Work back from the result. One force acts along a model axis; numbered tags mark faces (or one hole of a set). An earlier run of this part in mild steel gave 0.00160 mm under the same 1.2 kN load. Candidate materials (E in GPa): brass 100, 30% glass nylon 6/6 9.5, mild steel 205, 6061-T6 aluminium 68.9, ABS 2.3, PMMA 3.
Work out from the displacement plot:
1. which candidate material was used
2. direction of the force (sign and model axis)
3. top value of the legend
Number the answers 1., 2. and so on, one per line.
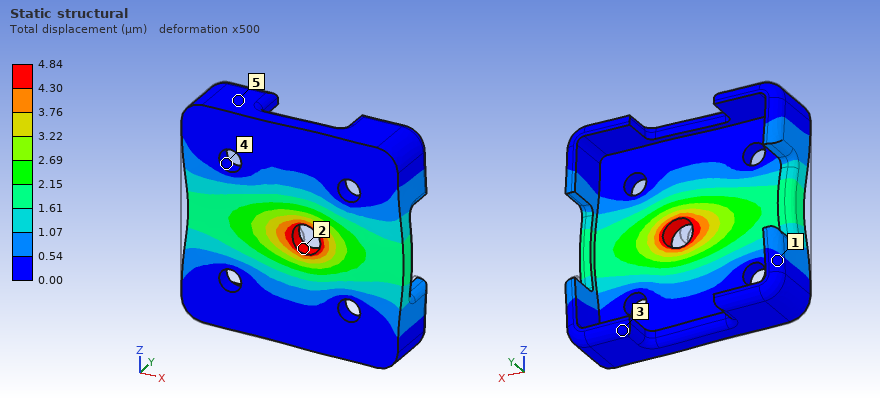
1. 6061-T6 aluminium
2. +X
3. 4.84 µm
